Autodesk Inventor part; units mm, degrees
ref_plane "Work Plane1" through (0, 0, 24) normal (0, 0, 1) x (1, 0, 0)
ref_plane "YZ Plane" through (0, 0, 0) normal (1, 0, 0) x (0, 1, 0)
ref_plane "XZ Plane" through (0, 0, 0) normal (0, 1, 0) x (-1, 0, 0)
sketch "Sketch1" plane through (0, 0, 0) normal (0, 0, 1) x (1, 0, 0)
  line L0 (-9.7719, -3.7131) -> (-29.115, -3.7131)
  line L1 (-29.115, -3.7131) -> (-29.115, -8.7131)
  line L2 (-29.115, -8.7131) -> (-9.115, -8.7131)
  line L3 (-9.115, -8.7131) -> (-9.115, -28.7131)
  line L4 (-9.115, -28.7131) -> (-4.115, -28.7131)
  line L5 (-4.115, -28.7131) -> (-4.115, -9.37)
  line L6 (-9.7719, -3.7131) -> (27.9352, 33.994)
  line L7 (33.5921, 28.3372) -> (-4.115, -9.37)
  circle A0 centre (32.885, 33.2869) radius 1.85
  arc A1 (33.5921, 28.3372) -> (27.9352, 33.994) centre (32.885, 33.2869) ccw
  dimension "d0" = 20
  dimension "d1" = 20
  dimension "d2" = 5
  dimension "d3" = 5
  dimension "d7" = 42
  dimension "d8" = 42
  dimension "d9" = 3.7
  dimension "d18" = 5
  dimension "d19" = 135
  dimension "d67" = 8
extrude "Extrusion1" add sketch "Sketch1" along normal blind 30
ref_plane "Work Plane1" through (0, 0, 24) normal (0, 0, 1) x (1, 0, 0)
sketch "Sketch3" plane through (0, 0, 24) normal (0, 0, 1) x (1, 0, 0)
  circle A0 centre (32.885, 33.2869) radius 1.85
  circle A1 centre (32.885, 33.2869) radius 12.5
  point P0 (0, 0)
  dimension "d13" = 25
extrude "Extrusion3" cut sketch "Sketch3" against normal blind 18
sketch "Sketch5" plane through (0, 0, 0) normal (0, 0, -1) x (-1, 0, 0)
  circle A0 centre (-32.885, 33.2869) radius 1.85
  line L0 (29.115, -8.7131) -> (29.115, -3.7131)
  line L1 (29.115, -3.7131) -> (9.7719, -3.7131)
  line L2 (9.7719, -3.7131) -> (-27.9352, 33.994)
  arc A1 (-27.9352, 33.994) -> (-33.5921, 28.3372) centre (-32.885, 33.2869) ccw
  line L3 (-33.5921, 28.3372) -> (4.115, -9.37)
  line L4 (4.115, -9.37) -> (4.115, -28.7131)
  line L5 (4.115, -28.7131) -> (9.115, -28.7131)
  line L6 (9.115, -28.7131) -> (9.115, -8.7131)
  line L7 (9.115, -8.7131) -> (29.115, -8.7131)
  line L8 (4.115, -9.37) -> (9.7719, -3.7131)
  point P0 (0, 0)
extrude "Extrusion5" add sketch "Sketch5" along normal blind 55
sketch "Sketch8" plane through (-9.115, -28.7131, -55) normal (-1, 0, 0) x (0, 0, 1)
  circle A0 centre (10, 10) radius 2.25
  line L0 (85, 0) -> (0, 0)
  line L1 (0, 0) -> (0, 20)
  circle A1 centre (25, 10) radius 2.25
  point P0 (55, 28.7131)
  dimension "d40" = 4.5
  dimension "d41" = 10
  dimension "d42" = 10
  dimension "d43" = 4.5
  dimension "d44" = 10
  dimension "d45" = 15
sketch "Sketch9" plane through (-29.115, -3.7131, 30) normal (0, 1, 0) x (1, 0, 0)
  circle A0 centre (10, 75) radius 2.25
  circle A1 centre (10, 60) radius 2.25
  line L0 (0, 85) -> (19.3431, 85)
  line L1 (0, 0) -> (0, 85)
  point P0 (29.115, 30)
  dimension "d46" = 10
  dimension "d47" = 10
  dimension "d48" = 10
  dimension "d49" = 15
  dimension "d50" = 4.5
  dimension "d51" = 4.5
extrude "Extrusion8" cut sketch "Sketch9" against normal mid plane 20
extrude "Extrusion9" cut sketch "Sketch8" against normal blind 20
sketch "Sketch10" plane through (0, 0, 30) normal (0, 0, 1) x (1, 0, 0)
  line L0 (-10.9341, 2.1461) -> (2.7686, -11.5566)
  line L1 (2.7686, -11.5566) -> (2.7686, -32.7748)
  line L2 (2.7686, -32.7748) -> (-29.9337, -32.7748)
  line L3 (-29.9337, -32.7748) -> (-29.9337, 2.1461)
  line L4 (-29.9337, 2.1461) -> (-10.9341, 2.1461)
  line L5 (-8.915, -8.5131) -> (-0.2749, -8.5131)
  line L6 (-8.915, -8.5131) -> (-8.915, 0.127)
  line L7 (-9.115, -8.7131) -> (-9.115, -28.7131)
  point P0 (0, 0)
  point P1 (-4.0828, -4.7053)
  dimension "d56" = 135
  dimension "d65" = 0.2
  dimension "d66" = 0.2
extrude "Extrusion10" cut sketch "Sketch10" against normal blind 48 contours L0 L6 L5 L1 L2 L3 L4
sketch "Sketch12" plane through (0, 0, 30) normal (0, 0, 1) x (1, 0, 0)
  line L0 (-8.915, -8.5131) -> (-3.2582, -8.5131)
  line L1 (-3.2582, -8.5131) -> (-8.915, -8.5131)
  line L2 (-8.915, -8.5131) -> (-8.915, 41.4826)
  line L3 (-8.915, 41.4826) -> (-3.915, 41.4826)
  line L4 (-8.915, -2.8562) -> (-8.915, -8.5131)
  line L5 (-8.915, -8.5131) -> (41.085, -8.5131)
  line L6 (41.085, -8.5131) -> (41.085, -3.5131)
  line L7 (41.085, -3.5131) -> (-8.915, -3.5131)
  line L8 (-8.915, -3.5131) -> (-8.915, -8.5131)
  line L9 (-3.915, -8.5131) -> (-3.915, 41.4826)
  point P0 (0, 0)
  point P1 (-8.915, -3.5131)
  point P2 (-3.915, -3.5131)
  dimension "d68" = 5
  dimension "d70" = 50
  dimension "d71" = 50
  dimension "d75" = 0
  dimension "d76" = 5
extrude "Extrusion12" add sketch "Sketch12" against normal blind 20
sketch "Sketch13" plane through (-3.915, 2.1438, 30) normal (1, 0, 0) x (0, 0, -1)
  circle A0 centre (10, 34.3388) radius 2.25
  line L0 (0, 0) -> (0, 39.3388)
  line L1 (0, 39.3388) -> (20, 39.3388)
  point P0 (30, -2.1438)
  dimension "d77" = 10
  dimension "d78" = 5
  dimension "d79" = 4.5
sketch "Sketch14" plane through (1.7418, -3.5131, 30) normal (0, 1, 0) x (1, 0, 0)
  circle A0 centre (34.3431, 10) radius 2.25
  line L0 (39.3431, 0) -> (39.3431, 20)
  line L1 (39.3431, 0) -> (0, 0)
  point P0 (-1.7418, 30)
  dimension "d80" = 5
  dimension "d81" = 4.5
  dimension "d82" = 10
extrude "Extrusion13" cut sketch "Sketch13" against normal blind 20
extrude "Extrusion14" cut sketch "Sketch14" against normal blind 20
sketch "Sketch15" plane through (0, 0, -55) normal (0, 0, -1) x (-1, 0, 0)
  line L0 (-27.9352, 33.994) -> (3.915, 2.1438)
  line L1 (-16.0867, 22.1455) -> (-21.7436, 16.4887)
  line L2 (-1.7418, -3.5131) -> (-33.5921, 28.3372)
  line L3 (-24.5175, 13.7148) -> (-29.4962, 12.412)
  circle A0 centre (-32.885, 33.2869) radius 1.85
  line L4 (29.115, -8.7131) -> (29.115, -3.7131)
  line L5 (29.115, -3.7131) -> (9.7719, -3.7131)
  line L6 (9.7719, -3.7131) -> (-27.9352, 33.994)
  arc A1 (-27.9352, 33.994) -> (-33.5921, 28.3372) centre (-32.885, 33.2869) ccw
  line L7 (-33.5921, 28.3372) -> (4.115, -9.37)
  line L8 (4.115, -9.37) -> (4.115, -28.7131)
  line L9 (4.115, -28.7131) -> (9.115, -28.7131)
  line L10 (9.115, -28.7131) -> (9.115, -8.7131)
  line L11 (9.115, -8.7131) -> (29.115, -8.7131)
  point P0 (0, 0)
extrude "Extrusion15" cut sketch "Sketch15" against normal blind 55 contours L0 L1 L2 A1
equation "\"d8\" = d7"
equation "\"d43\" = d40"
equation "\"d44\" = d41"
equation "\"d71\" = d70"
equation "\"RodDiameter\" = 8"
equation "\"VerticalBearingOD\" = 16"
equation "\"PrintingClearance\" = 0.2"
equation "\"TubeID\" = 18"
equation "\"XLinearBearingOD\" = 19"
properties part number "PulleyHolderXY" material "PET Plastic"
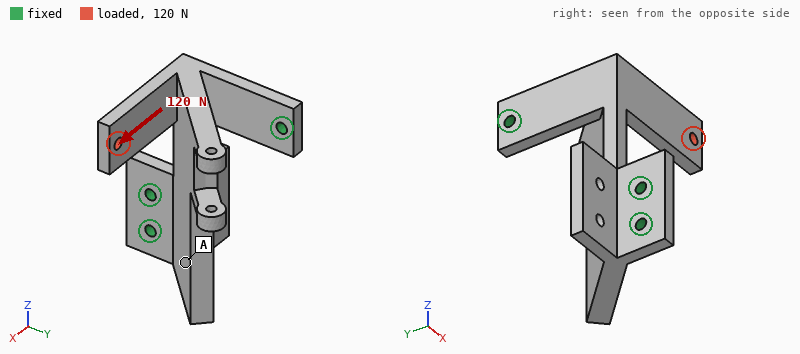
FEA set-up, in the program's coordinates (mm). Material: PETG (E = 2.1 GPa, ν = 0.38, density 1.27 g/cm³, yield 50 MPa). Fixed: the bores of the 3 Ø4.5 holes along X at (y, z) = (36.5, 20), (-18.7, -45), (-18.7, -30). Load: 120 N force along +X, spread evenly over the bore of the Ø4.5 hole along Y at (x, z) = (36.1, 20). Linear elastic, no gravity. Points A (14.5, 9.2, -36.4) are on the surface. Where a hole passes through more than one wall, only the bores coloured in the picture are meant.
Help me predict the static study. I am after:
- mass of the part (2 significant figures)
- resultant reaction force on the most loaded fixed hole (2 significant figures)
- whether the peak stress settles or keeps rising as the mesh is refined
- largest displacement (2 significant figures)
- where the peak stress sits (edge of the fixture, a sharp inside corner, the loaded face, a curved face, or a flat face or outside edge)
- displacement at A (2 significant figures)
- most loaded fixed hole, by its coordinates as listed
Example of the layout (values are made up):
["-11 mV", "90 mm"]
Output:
["56 g", "320 N", "keeps rising", "1.5 mm", "edge of the fixture", "0.34 mm", "(-18.7, -30)"]
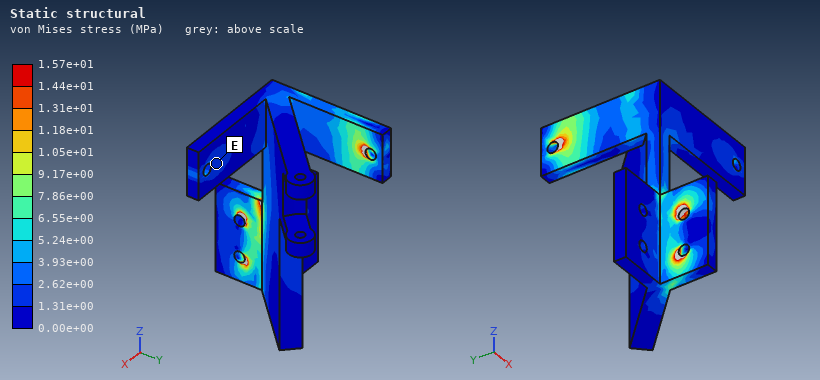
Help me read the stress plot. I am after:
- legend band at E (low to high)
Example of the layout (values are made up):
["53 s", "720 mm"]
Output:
["1.31e+00 to 2.62e+00 MPa"]
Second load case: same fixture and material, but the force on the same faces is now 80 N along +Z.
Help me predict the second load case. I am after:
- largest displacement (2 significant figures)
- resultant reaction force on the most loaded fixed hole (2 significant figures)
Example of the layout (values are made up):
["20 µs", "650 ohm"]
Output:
["1.3 mm", "240 N"]
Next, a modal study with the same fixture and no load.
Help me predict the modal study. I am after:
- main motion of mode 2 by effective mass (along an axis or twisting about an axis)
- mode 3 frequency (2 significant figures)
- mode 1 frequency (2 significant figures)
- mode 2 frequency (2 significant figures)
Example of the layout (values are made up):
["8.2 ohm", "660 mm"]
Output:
["along X", "600 Hz", "320 Hz", "400 Hz"]
